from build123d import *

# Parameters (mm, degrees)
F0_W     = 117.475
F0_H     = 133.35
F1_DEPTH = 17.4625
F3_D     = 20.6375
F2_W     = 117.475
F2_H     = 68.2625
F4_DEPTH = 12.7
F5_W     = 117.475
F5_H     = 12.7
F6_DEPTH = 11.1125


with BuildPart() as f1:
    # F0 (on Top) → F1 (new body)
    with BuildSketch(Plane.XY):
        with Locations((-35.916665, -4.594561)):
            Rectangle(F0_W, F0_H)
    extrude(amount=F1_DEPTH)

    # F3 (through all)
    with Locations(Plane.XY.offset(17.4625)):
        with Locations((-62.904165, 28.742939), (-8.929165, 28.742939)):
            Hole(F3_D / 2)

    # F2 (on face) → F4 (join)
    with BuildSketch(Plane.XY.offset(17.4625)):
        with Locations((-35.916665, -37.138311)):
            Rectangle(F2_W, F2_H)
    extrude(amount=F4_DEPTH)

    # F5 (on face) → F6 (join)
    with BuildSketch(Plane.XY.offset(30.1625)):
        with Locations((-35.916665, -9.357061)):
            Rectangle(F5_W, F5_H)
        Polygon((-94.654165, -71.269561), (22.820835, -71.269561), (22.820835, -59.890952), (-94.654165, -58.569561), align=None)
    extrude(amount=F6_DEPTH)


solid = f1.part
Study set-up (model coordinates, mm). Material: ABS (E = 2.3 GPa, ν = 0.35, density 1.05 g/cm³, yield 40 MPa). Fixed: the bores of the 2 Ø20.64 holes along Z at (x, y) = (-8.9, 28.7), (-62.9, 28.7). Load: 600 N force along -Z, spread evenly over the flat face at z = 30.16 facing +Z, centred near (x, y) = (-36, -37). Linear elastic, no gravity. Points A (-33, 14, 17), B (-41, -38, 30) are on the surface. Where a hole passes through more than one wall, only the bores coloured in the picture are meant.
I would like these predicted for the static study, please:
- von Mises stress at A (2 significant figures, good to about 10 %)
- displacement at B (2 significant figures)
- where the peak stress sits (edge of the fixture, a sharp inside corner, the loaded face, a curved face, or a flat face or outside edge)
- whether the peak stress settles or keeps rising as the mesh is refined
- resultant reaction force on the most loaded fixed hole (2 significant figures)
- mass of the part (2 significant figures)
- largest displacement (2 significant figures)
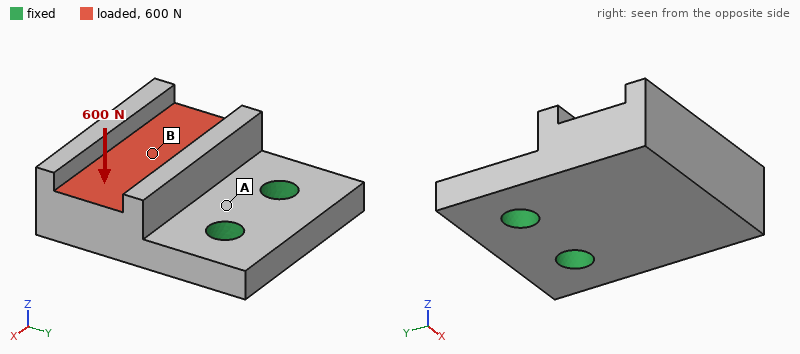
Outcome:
3.5 MPa
0.39 mm
edge of the fixture
keeps rising
300 N
420 g
0.66 mm
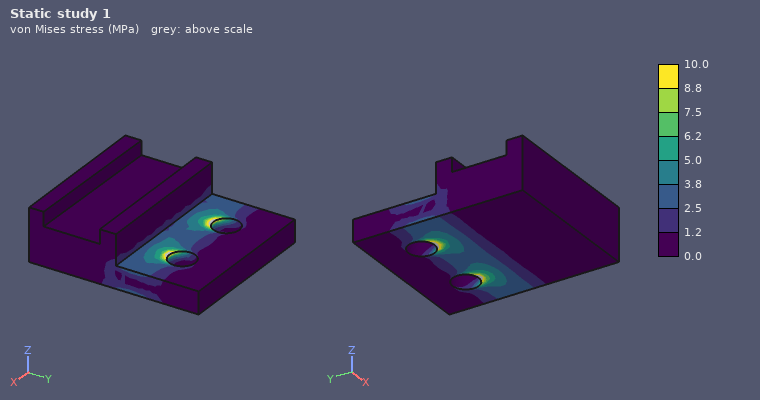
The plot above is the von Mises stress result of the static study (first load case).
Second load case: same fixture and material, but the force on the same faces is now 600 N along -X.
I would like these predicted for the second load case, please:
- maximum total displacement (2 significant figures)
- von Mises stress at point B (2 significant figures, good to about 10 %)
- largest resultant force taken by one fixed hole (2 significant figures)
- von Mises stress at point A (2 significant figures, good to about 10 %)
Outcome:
97 µm
0.61 MPa
630 N
0.99 MPa
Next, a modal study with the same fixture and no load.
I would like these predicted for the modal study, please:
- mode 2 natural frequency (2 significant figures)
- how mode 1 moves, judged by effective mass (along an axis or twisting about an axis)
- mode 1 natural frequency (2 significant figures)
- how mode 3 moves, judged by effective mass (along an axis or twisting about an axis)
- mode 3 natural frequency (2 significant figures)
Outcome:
860 Hz
along Z
340 Hz
along X
1100 Hz
